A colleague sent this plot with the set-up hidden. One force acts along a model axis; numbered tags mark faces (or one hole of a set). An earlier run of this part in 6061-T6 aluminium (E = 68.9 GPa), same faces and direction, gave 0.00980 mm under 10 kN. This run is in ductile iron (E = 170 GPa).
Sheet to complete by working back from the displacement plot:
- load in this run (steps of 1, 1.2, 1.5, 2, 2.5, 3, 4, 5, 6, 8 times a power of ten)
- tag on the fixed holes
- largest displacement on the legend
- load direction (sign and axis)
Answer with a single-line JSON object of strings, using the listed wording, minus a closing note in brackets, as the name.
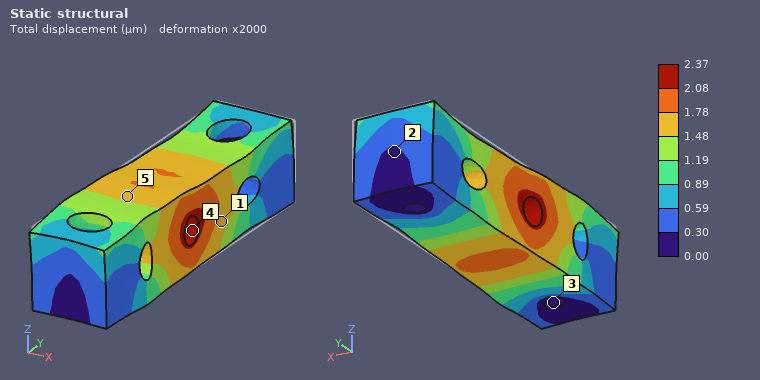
{"load in this run": "6 kN", "tag on the fixed holes": "3", "largest displacement on the legend": "2.37 µm", "load direction": "-Y"}
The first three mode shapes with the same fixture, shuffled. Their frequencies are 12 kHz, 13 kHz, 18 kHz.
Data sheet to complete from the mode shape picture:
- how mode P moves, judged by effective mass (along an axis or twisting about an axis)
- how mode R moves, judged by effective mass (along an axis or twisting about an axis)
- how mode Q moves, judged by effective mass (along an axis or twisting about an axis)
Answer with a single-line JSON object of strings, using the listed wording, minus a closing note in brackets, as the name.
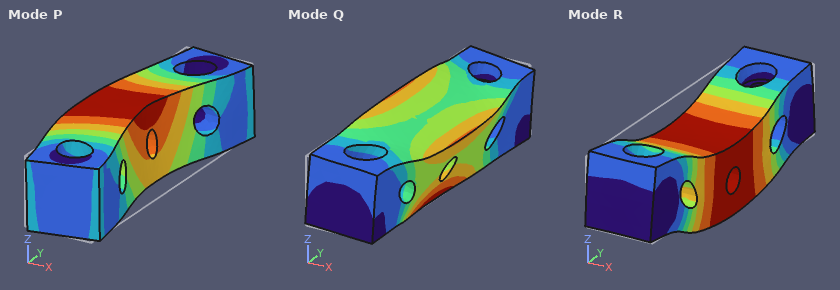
{"how mode P moves, judged by effective mass": "along X", "how mode R moves, judged by effective mass": "along Z", "how mode Q moves, judged by effective mass": "twisting about Y"}
